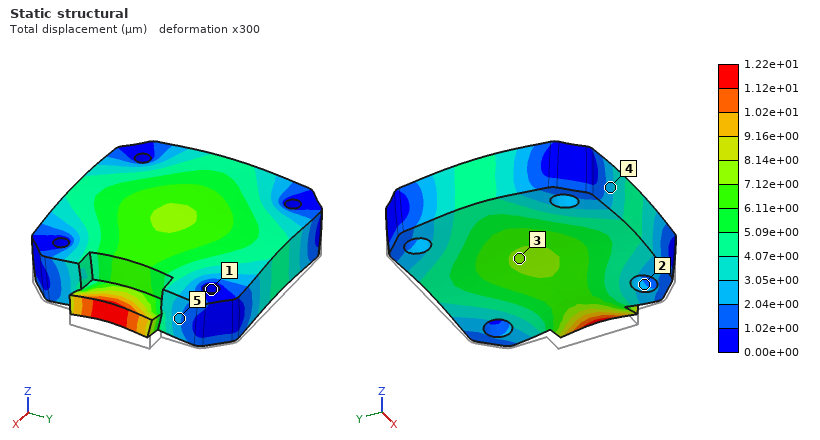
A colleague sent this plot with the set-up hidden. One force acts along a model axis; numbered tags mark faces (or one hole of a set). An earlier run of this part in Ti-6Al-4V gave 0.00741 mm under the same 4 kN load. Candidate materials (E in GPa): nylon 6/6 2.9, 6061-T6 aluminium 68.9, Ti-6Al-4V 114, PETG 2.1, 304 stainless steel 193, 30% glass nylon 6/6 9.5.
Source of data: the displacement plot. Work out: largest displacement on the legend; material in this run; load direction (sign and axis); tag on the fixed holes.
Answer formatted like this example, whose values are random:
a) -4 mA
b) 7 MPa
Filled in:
a) 1.22e+01 µm
b) 6061-T6 aluminium
c) +Z
d) 1
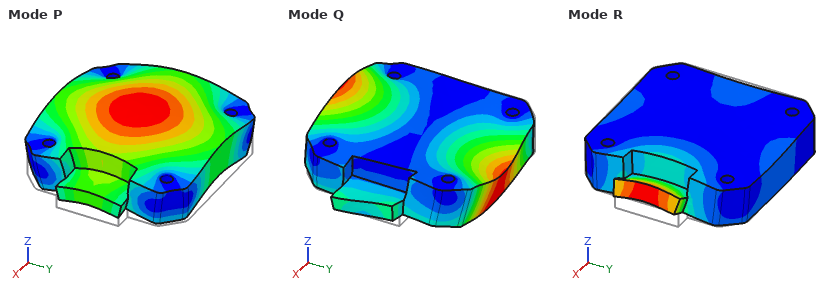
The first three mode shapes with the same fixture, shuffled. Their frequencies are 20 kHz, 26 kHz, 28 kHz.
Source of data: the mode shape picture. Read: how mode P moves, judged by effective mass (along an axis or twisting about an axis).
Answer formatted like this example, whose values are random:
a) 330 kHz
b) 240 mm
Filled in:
a) along Z
